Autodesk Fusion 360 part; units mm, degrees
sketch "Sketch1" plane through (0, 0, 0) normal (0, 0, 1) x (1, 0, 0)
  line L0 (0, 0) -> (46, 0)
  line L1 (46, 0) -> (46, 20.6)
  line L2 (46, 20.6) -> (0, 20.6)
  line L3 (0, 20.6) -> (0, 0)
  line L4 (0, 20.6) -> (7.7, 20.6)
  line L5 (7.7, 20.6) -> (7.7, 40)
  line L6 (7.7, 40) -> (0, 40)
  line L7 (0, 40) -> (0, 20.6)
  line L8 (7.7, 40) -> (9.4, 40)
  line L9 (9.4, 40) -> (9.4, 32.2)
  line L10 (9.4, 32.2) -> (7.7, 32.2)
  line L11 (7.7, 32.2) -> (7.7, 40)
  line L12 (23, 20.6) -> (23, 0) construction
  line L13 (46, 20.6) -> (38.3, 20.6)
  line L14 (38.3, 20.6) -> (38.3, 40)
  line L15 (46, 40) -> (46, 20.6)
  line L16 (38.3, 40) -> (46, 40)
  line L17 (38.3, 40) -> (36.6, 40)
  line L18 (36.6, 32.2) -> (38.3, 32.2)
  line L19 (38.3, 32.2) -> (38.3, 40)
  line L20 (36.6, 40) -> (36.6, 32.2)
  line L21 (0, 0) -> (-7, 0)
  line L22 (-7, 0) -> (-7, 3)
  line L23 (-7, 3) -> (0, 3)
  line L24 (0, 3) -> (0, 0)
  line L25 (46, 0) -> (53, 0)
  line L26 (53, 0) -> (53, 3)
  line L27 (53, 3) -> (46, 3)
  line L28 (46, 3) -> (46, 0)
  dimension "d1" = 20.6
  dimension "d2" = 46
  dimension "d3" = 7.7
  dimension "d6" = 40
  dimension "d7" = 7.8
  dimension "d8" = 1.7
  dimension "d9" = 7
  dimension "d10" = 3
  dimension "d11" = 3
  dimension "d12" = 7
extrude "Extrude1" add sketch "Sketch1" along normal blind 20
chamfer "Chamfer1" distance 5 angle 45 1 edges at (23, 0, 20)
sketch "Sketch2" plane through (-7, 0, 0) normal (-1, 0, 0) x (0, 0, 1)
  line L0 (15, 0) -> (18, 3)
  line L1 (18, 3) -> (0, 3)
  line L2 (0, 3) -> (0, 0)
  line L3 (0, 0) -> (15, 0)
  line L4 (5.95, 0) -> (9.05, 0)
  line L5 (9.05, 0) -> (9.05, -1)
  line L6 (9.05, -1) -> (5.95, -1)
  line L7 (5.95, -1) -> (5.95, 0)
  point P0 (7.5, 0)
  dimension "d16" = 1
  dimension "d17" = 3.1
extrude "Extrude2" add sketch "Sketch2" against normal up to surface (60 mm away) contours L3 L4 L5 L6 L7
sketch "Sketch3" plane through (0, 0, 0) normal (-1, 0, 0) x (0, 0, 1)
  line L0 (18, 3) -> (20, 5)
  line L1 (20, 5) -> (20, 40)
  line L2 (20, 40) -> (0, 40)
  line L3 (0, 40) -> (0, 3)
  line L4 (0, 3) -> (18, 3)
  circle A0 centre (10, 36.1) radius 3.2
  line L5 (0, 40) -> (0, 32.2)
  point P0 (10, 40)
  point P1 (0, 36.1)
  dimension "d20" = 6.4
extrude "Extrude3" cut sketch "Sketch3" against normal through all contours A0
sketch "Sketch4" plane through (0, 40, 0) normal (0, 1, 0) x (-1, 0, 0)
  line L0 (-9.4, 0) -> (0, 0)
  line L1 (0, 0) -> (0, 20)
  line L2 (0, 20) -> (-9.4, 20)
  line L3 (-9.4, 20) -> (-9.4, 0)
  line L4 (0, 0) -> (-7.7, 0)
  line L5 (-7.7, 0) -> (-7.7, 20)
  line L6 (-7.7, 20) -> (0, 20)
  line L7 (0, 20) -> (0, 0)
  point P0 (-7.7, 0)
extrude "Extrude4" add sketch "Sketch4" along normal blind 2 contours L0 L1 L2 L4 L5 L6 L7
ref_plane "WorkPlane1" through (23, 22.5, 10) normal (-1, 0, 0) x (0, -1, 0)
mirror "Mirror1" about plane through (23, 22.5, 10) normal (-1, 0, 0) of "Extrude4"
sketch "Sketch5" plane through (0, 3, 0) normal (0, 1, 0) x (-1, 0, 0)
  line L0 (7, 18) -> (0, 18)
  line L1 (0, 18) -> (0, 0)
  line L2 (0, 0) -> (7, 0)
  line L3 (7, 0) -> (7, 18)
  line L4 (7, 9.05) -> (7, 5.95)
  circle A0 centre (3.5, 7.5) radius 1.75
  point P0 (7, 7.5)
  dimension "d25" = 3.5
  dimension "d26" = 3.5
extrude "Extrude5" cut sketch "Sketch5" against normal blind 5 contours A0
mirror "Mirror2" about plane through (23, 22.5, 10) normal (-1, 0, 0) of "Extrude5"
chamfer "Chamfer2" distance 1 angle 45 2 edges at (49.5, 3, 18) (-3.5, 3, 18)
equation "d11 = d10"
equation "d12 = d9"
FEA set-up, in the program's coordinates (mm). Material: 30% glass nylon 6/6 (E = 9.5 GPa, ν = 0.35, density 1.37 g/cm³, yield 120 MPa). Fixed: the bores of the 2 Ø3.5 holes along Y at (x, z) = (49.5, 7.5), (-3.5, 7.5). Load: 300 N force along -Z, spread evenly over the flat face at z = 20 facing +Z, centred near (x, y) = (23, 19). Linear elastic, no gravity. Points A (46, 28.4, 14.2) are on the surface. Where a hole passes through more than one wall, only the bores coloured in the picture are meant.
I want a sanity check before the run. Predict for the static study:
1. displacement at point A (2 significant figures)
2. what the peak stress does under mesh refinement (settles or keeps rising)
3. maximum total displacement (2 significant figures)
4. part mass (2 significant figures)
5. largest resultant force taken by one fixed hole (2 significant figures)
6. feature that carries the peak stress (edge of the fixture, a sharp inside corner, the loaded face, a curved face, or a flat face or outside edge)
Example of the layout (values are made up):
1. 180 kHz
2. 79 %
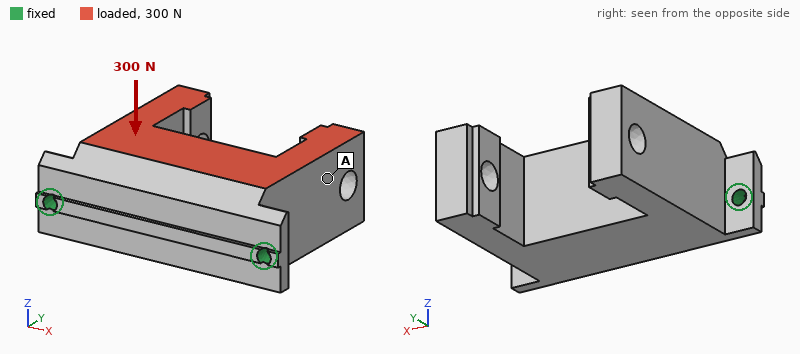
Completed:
1. 0.48 mm
2. keeps rising
3. 0.74 mm
4. 35 g
5. 150 N
6. edge of the fixture
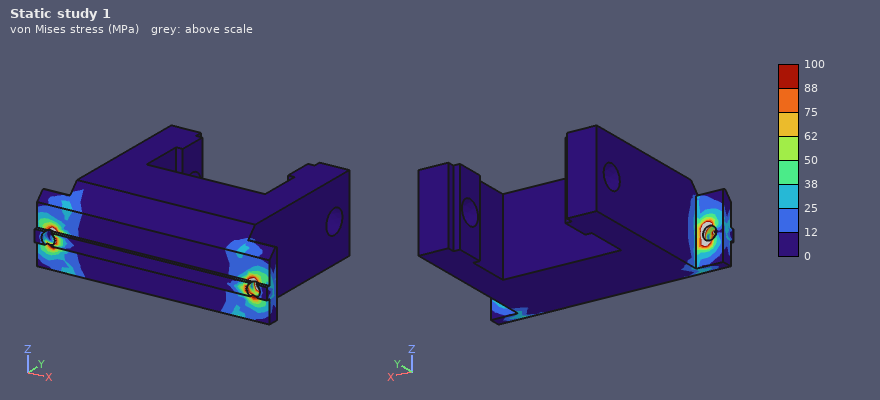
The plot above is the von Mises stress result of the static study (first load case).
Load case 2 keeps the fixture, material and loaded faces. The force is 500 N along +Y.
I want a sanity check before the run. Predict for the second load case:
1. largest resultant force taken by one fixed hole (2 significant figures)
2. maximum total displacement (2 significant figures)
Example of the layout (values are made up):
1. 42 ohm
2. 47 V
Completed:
1. 280 N
2. 0.86 mm
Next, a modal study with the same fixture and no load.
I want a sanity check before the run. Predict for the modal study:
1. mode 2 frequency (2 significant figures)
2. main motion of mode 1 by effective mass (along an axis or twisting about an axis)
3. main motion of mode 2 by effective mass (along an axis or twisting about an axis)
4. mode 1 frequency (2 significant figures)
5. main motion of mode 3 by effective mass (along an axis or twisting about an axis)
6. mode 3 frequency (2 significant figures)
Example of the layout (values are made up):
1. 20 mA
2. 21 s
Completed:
1. 3600 Hz
2. along Z
3. along X
4. 780 Hz
5. along Y
6. 4300 Hz
